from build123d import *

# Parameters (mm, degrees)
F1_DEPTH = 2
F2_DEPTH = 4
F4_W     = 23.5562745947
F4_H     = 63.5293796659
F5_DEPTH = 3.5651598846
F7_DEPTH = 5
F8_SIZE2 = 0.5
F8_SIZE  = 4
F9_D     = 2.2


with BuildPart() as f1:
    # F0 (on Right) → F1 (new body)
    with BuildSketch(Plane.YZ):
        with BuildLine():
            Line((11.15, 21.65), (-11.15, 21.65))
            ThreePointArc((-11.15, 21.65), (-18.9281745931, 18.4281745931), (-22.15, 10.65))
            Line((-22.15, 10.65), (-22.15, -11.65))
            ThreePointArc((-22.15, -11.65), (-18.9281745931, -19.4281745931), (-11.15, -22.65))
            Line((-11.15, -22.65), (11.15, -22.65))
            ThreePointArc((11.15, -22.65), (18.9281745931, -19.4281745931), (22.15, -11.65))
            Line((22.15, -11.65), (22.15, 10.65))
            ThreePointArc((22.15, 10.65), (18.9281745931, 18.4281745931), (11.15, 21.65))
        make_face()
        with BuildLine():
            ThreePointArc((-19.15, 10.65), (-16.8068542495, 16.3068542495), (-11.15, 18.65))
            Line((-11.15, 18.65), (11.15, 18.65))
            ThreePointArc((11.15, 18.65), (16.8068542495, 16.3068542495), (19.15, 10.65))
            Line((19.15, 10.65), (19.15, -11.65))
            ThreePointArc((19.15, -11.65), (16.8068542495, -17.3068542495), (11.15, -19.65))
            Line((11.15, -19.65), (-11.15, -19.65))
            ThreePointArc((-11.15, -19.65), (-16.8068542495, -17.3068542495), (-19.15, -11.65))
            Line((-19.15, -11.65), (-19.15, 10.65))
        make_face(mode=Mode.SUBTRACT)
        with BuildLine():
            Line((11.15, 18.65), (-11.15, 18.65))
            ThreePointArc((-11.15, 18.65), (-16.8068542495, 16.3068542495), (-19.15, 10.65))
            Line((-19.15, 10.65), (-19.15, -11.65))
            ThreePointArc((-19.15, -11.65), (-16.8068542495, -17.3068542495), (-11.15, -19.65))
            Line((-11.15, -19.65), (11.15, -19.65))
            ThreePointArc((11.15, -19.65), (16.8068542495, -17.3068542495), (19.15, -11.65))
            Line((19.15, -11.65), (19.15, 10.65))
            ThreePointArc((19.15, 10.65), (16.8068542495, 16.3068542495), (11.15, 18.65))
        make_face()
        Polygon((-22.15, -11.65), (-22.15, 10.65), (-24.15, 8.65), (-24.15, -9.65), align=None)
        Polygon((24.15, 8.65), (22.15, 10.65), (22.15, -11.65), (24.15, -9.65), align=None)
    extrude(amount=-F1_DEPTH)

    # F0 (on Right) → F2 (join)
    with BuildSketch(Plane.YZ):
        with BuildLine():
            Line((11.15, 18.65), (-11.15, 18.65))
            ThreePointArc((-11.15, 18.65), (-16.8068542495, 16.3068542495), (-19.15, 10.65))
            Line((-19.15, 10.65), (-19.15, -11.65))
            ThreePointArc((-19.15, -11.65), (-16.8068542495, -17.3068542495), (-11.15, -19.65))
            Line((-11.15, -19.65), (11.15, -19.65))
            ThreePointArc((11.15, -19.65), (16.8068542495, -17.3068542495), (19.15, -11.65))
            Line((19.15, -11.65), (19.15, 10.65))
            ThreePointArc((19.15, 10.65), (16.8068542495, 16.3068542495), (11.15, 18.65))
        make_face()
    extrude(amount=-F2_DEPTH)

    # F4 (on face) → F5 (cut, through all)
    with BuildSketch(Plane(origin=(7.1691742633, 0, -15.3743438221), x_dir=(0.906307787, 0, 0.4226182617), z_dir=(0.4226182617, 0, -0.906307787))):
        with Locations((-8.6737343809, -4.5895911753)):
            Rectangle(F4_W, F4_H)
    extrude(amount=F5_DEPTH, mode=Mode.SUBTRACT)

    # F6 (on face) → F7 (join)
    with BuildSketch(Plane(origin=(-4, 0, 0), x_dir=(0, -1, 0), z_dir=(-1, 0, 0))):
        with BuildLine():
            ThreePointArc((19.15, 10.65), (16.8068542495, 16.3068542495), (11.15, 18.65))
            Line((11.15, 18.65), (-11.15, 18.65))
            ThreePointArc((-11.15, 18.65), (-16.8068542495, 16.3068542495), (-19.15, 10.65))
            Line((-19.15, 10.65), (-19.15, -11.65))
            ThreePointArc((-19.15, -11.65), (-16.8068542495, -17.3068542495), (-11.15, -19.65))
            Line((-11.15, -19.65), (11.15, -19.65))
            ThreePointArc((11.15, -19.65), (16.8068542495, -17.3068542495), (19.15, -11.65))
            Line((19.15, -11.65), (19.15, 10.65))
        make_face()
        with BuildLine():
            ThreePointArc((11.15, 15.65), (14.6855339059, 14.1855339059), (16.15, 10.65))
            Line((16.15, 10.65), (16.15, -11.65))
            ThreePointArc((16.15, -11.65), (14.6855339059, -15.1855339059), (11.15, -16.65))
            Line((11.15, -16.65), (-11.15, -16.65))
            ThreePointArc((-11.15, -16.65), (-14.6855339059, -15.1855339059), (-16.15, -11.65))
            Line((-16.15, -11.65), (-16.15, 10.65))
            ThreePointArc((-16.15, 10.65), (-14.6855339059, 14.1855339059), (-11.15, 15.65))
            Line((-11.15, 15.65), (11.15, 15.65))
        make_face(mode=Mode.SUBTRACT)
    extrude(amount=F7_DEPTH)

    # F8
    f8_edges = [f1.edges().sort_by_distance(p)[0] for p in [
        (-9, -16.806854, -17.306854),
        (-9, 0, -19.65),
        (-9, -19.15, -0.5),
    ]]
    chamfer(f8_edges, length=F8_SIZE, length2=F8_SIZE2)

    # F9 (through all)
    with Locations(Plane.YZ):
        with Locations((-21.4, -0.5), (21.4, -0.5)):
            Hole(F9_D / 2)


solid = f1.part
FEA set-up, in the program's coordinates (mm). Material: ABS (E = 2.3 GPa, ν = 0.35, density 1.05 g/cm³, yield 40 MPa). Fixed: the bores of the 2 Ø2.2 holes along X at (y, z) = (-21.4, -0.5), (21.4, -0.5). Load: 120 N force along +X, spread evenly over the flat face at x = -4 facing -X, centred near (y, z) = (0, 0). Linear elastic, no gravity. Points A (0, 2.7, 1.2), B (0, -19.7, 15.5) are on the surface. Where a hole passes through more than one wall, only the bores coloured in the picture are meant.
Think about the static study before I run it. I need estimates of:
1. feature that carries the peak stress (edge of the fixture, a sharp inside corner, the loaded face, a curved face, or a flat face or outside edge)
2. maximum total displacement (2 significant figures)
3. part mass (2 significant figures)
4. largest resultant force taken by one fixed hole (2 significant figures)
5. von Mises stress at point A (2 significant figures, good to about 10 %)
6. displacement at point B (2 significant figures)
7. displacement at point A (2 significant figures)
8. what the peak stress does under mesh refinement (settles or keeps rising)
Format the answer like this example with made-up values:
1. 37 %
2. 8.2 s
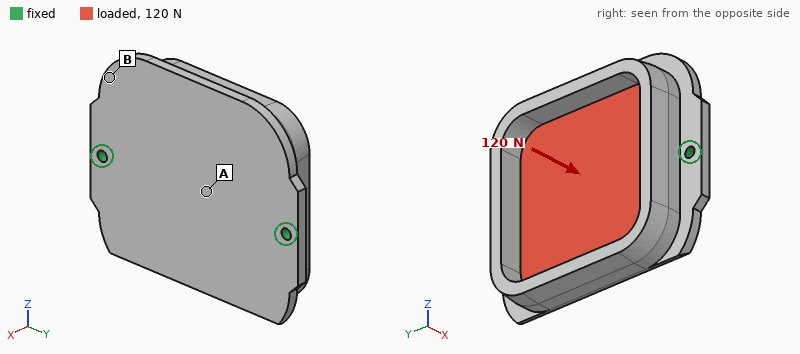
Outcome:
1. edge of the fixture
2. 0.14 mm
3. 8.7 g
4. 79 N
5. 2.4 MPa
6. 0.071 mm
7. 0.13 mm
8. keeps rising
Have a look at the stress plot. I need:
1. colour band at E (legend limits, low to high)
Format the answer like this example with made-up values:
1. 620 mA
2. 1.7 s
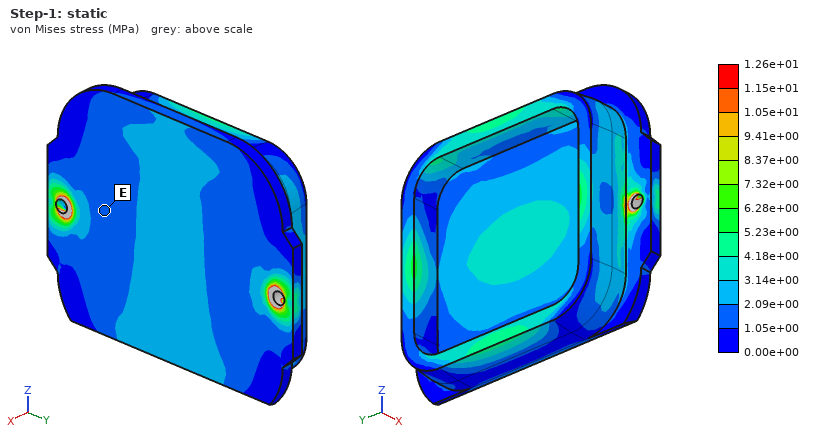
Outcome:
1. 1.05e+00 to 2.09e+00 MPa
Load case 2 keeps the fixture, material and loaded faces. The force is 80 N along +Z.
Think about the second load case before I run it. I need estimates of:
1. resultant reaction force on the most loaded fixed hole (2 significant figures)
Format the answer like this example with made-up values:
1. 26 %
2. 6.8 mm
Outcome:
1. 40 N
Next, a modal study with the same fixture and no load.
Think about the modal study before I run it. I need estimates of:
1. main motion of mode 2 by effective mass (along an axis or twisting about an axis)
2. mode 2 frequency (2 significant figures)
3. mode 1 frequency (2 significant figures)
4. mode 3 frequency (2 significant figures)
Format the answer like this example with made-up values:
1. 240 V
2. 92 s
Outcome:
1. along X
2. 1800 Hz
3. 650 Hz
4. 2500 Hz
